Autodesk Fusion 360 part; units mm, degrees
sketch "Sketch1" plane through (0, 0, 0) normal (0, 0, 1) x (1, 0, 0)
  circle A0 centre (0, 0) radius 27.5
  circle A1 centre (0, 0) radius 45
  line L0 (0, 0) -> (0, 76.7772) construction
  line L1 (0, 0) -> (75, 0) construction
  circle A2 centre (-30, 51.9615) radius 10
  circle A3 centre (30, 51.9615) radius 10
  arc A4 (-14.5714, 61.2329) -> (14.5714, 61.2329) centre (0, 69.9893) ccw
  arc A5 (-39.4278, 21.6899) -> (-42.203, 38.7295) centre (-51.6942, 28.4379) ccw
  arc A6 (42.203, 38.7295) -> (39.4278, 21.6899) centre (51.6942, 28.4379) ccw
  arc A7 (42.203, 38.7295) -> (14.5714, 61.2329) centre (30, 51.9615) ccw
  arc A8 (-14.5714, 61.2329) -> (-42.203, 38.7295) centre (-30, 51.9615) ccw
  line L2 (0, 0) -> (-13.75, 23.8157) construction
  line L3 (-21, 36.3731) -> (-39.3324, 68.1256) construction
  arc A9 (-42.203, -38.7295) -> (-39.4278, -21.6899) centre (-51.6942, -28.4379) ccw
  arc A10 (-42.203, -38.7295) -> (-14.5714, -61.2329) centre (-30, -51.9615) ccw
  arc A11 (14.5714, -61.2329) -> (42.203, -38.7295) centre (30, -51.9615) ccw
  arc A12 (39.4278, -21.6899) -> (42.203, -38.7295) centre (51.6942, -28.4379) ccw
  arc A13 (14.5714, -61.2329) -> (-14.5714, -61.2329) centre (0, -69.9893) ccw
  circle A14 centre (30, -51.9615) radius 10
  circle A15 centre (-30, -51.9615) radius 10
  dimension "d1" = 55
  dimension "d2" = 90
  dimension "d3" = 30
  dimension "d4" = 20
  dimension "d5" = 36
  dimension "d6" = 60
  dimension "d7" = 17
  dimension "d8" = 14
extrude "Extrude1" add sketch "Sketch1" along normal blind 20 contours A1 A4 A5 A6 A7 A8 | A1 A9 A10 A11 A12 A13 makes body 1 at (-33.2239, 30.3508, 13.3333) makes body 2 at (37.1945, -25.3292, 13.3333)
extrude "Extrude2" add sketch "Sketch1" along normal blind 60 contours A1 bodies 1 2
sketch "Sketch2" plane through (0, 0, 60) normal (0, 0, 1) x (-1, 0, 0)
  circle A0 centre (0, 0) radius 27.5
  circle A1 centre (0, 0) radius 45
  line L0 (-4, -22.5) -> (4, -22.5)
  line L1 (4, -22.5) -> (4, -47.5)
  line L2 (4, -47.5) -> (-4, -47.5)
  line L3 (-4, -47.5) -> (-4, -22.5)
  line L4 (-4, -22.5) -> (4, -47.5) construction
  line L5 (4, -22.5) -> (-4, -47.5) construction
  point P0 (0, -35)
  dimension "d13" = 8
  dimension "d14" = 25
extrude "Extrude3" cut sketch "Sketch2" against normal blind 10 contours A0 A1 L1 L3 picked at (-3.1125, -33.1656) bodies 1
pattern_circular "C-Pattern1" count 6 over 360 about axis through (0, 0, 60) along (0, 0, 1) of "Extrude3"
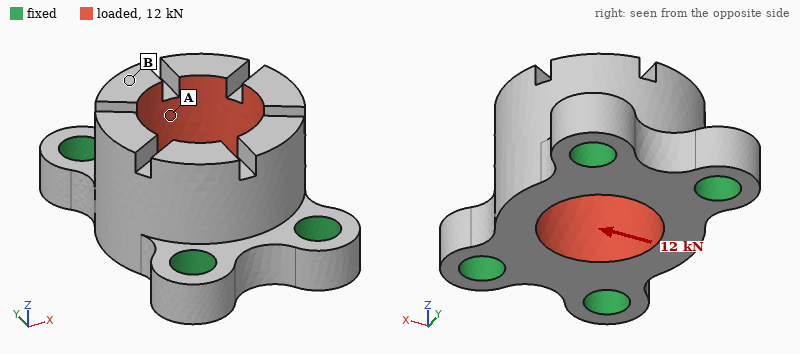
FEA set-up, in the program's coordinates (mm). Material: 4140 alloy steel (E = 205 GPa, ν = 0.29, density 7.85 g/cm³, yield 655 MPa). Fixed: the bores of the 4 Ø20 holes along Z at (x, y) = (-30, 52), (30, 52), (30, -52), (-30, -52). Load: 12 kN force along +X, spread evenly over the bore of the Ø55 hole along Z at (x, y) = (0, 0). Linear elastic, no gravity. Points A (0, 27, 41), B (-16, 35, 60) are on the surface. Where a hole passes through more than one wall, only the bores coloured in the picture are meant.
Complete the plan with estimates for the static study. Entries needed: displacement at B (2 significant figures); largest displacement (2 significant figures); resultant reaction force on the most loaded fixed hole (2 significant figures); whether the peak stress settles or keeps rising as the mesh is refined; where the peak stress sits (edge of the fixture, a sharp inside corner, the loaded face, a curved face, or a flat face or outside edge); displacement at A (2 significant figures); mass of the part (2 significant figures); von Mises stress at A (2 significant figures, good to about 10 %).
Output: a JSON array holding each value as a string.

["3.4 µm", "5.0 µm", "3.7 kN", "keeps rising", "edge of the fixture", "2.4 µm", "2.3 kg", "6.7 MPa"]
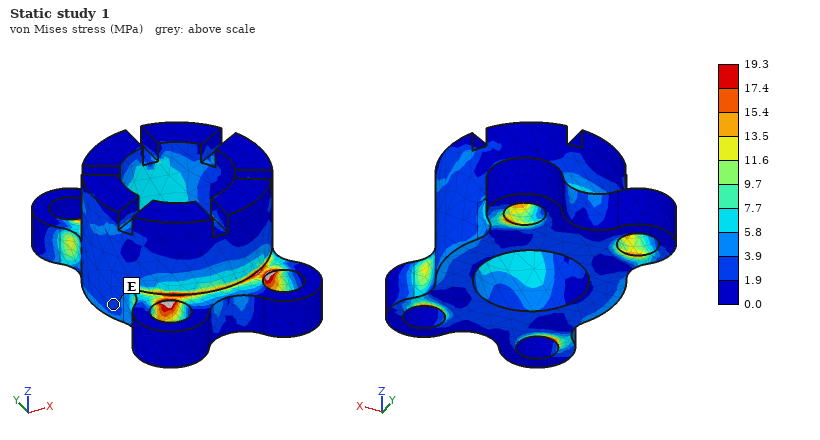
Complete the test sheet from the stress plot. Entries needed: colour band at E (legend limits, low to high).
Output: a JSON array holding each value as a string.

["1.9 to 3.9 MPa"]
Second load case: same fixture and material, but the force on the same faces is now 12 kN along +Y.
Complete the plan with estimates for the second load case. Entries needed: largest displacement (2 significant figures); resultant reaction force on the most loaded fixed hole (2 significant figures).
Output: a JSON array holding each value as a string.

["2.7 µm", "3.3 kN"]
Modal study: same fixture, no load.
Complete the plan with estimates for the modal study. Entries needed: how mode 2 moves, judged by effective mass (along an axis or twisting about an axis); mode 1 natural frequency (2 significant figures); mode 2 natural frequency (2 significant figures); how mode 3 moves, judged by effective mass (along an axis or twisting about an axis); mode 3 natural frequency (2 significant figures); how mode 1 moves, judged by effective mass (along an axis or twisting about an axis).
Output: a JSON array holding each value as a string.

["along Z", "6800 Hz", "7900 Hz", "along Y", "10 kHz", "along X"]
